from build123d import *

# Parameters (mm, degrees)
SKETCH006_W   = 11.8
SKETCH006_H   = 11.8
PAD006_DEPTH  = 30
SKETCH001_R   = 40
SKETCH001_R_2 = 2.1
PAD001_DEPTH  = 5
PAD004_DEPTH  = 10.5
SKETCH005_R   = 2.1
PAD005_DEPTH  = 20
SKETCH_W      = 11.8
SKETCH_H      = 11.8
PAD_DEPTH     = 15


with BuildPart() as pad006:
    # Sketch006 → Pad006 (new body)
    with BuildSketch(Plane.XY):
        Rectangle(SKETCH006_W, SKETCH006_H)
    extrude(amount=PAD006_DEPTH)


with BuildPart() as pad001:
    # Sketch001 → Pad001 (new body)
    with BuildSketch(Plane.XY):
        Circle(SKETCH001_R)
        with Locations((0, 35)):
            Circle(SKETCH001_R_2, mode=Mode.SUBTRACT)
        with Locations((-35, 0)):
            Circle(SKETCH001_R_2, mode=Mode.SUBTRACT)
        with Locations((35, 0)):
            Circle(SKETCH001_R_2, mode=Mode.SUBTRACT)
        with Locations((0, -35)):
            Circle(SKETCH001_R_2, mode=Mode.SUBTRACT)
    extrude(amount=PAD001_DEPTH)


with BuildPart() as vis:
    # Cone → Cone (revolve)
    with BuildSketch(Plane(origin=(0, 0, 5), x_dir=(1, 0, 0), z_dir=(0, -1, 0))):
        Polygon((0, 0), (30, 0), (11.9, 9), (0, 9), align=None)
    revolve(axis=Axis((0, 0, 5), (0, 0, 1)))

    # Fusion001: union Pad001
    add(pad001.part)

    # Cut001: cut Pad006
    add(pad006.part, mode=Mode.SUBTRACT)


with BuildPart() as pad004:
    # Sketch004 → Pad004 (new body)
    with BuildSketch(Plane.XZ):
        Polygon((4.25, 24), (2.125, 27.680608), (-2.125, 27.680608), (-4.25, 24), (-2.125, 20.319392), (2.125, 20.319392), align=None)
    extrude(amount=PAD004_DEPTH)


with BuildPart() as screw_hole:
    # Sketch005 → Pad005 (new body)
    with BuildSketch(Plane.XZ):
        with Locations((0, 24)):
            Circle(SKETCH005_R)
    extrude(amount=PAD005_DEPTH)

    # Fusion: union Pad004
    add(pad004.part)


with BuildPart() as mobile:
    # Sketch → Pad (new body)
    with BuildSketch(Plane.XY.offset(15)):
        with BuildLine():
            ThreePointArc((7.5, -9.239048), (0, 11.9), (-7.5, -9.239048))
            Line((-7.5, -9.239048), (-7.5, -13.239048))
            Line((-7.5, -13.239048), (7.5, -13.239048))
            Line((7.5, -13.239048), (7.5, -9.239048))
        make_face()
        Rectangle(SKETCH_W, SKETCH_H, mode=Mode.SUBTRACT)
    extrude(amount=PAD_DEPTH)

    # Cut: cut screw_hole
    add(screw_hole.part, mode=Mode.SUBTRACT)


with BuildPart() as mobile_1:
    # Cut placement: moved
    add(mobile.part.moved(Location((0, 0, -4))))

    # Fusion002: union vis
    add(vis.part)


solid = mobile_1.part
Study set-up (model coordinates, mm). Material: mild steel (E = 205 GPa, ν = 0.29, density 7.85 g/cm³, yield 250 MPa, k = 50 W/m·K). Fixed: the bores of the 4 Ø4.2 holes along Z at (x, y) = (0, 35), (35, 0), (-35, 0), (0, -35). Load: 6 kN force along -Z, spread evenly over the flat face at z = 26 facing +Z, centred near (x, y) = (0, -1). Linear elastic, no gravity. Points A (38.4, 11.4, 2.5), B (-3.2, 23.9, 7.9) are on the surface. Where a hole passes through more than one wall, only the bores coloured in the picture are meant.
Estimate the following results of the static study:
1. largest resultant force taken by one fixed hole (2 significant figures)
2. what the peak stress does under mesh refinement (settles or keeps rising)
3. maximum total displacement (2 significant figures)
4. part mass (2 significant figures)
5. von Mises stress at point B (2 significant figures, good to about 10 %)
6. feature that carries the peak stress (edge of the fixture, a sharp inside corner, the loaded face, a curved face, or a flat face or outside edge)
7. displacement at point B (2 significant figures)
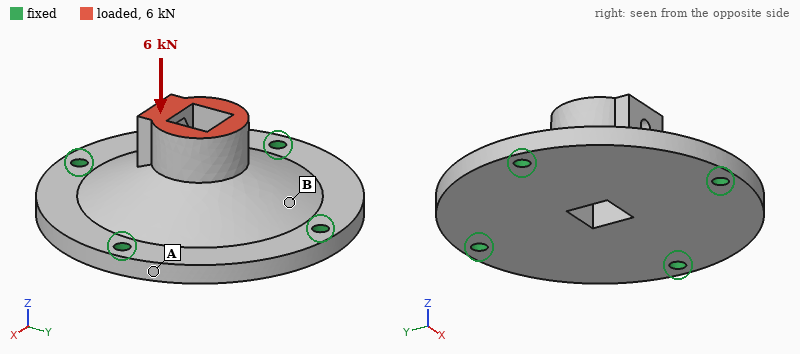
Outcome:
2.1 kN
keeps rising
14 µm
310 g
37 MPa
edge of the fixture
6.8 µm
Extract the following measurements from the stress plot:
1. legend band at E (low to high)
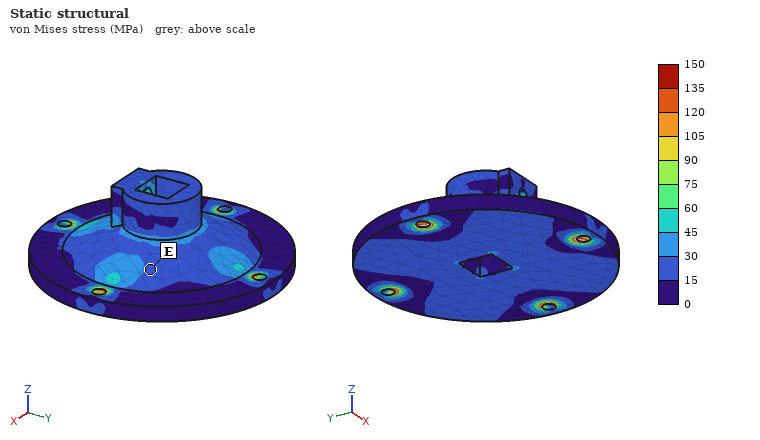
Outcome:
15 to 30 MPa
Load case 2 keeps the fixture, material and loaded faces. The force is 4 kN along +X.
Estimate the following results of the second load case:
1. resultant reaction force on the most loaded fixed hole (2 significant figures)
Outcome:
2.2 kN
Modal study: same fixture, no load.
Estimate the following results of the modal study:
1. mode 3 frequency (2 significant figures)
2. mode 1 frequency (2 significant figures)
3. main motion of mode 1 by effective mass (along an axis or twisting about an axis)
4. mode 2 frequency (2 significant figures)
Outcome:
10 kHz
8200 Hz
along Z
10 kHz
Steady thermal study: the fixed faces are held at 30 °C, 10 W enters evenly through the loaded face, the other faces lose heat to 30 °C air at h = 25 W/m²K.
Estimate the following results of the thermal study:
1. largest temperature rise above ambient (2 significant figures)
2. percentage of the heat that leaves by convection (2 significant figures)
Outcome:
18 K
16 %
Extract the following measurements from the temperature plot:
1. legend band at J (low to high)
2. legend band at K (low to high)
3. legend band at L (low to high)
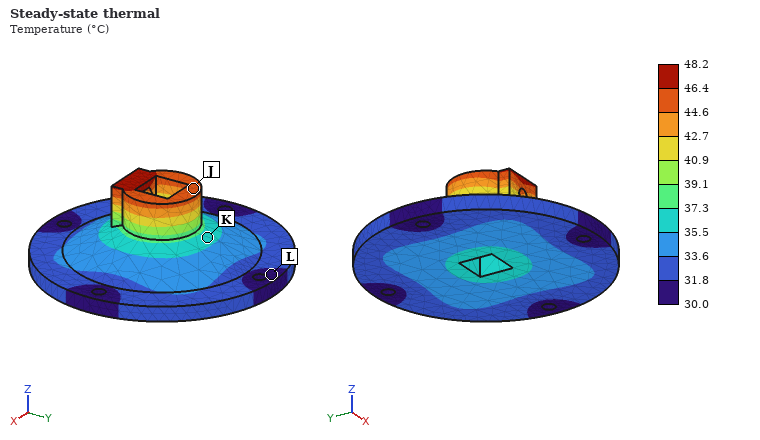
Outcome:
44.6 to 46.4 °C
35.5 to 37.3 °C
30.0 to 31.8 °C
